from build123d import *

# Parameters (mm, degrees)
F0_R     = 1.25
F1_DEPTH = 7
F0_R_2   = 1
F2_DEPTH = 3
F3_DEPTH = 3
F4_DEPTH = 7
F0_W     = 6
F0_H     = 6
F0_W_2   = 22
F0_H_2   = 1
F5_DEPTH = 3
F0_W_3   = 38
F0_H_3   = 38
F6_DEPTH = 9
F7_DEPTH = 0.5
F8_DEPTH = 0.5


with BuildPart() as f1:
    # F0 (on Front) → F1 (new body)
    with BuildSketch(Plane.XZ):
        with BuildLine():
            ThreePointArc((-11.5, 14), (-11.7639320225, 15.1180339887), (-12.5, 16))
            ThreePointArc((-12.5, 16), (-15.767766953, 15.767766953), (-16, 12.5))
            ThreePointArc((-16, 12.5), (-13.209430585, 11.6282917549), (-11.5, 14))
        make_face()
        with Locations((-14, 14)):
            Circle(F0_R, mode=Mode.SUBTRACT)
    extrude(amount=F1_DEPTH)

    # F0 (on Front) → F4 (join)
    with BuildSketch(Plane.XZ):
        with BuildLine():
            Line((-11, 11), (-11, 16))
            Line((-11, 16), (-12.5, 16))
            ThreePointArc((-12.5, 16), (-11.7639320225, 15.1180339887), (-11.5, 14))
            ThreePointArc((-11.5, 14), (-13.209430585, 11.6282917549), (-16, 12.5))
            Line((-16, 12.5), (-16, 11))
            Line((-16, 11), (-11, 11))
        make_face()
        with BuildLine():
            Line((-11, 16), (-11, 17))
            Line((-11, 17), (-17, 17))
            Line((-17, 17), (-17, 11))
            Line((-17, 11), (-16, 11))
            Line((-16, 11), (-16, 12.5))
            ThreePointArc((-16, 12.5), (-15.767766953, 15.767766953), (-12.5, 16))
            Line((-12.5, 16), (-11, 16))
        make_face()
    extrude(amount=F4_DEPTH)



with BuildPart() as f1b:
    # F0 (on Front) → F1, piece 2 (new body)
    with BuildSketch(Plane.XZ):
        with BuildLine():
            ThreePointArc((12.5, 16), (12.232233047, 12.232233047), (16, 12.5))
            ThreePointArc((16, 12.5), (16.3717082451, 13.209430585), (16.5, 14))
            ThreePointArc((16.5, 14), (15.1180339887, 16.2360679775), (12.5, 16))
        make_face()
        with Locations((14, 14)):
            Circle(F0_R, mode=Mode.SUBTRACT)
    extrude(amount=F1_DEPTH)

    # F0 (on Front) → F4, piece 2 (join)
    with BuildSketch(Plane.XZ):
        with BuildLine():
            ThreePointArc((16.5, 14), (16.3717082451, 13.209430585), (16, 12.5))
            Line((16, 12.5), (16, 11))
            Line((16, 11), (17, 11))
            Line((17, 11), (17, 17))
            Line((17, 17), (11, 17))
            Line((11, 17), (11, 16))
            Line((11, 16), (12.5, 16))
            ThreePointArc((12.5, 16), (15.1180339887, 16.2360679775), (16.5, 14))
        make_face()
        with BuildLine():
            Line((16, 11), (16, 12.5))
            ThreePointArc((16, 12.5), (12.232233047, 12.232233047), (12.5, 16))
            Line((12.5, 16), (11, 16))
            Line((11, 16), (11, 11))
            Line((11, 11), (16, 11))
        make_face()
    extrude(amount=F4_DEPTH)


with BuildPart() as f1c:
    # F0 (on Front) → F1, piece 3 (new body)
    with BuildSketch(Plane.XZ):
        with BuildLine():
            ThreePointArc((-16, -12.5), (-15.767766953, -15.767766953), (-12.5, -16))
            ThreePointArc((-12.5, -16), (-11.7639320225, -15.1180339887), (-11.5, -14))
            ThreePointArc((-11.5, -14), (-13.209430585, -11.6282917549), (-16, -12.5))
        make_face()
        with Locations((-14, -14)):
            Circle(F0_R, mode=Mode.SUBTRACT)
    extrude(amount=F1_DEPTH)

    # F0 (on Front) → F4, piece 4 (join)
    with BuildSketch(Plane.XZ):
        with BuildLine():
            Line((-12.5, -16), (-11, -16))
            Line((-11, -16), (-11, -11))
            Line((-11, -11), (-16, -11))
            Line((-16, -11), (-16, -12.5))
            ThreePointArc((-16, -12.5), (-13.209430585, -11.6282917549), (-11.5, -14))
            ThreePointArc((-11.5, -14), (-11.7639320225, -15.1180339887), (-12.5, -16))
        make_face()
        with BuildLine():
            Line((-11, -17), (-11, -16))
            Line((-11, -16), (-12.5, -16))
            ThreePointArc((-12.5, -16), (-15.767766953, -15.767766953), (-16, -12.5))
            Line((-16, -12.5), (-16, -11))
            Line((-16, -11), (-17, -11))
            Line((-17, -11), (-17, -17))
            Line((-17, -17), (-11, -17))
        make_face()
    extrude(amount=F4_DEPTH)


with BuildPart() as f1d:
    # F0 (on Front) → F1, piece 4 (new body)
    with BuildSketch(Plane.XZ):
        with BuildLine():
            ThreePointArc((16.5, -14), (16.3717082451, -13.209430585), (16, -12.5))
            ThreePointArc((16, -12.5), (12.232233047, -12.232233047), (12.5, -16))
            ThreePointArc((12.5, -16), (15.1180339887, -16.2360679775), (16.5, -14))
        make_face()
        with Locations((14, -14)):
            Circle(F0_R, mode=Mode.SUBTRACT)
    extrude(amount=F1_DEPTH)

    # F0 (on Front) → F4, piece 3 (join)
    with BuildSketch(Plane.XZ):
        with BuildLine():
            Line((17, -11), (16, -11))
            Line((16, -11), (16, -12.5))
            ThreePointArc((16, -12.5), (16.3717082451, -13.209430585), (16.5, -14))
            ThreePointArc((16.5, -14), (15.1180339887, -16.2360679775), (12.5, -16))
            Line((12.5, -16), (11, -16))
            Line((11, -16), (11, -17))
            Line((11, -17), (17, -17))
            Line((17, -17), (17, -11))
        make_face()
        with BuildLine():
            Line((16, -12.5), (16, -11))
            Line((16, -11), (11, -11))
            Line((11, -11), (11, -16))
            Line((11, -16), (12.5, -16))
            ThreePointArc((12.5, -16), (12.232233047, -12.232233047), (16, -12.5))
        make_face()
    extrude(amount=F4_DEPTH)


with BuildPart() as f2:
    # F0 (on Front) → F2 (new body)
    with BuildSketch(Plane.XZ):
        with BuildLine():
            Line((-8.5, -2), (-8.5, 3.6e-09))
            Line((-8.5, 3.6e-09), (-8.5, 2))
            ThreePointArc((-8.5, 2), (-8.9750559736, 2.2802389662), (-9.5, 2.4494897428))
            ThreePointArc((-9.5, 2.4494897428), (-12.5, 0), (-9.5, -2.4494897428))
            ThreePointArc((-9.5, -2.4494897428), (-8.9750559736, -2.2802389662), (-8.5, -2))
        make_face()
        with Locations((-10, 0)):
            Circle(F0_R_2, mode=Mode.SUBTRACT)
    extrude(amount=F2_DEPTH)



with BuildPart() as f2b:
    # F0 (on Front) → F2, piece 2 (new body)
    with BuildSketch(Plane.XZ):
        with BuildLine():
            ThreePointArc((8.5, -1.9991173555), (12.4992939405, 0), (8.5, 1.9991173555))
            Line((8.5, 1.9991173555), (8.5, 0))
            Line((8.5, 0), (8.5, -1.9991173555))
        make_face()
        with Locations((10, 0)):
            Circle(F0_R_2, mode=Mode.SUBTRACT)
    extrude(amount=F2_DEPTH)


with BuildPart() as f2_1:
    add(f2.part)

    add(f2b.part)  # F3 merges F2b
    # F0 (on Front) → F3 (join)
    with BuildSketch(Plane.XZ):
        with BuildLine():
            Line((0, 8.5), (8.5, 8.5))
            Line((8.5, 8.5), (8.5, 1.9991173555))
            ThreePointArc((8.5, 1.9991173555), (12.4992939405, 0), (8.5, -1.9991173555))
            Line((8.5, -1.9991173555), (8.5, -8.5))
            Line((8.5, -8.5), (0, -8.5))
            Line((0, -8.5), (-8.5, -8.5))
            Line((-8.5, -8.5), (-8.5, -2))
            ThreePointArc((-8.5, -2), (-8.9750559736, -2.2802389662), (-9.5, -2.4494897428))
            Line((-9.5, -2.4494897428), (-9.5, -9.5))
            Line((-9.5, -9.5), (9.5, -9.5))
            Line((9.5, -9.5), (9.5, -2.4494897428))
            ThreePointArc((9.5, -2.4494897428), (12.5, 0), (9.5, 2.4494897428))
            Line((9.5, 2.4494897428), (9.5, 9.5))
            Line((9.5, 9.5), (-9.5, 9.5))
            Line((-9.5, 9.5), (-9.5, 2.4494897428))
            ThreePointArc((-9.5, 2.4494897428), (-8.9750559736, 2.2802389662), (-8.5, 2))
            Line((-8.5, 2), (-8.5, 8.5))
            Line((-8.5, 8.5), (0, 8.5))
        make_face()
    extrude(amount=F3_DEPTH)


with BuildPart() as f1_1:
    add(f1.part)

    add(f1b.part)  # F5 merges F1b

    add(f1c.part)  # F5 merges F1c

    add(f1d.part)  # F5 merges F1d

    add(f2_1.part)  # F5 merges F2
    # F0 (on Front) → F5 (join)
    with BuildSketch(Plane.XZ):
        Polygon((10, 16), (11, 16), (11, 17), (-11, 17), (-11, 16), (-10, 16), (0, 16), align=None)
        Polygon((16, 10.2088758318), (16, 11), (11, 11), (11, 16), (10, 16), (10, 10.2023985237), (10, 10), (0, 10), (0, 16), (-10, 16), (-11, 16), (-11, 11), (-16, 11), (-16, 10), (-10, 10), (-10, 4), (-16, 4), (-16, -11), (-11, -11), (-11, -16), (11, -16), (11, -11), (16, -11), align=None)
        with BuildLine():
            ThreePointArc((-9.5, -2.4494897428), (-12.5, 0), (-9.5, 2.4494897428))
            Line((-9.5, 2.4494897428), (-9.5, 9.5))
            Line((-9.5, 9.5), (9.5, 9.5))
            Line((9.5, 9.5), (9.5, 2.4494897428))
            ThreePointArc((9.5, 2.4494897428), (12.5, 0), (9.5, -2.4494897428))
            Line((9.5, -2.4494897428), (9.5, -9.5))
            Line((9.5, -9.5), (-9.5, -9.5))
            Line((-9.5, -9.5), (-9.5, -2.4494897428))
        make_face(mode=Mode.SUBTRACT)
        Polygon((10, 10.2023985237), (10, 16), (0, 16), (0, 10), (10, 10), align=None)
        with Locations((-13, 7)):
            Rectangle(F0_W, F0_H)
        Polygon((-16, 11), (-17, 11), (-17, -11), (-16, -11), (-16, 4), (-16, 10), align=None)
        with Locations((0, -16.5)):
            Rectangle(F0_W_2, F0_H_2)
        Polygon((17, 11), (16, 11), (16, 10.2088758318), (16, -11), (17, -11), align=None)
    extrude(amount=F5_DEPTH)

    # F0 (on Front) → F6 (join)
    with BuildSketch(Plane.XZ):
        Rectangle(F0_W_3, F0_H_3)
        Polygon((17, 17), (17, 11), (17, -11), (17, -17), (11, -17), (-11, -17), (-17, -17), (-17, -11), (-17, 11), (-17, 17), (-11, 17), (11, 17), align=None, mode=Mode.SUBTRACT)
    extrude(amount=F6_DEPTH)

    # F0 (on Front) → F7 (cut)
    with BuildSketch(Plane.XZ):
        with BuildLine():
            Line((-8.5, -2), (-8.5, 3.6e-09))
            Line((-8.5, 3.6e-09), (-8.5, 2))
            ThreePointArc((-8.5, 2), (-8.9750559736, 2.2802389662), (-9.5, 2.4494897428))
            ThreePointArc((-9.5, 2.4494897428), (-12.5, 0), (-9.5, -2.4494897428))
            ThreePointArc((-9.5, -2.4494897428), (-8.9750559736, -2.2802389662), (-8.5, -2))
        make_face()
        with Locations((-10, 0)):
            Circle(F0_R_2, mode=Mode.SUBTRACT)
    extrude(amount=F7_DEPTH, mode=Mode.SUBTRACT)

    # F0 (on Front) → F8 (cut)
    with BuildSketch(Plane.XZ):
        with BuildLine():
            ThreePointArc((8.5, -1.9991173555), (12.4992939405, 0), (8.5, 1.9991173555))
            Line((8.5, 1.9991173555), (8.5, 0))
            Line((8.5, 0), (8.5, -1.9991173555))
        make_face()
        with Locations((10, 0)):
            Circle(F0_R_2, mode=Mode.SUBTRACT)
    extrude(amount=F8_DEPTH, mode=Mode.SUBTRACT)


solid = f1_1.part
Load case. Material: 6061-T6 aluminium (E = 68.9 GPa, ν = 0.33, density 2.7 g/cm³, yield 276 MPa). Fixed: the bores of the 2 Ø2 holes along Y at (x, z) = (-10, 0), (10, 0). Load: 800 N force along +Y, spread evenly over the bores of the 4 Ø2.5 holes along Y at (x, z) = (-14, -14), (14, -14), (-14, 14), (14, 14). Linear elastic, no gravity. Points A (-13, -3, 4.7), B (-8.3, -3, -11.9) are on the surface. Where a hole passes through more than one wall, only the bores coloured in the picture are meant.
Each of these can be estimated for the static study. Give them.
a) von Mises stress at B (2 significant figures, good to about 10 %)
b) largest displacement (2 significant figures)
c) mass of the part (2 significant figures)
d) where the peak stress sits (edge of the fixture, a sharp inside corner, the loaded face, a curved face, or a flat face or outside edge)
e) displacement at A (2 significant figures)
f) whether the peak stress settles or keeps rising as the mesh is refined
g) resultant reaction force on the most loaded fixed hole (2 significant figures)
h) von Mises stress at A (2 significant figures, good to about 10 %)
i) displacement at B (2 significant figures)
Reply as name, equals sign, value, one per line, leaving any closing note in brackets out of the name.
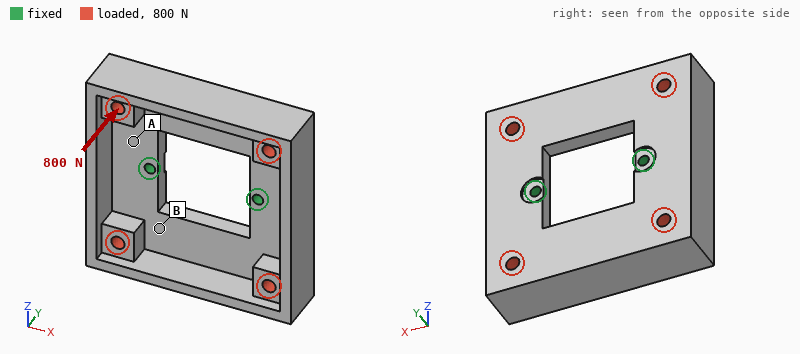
von Mises stress at B = 13 MPa
largest displacement = 42 µm
mass of the part = 15 g
where the peak stress sits = edge of the fixture
displacement at A = 13 µm
whether the peak stress settles or keeps rising as the mesh is refined = keeps rising
resultant reaction force on the most loaded fixed hole = 410 N
von Mises stress at A = 31 MPa
displacement at B = 26 µm
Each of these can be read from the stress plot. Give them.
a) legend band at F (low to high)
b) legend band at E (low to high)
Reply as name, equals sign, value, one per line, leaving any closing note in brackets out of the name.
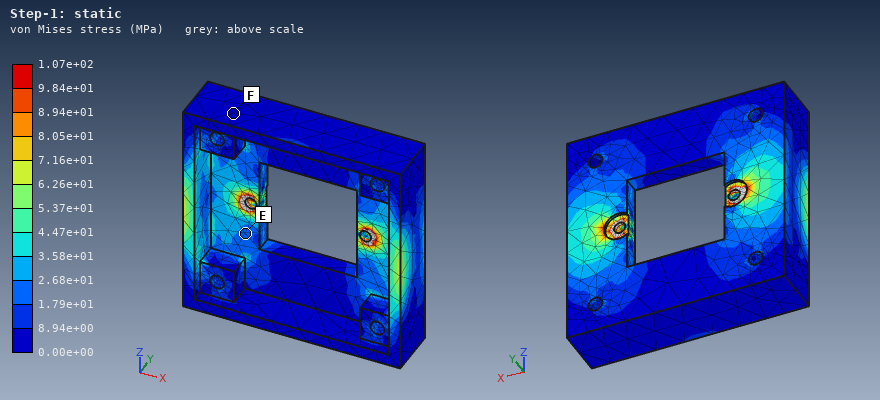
legend band at F = 0.00e+00 to 8.94e+00 MPa
legend band at E = 1.79e+01 to 2.68e+01 MPa
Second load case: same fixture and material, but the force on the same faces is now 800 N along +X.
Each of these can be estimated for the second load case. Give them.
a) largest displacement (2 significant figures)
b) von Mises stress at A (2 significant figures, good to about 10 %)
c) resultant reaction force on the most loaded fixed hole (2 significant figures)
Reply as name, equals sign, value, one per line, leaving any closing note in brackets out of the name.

largest displacement = 15 µm
von Mises stress at A = 18 MPa
resultant reaction force on the most loaded fixed hole = 400 N
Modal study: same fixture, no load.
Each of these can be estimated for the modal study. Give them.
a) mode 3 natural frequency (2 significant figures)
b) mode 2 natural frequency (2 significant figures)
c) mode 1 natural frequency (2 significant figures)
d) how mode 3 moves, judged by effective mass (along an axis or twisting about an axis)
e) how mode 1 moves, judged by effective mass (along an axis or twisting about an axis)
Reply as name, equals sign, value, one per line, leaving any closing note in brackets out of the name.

mode 3 natural frequency = 6800 Hz
mode 2 natural frequency = 5300 Hz
mode 1 natural frequency = 2600 Hz
how mode 3 moves, judged by effective mass = along Y
how mode 1 moves, judged by effective mass = twisting about X
